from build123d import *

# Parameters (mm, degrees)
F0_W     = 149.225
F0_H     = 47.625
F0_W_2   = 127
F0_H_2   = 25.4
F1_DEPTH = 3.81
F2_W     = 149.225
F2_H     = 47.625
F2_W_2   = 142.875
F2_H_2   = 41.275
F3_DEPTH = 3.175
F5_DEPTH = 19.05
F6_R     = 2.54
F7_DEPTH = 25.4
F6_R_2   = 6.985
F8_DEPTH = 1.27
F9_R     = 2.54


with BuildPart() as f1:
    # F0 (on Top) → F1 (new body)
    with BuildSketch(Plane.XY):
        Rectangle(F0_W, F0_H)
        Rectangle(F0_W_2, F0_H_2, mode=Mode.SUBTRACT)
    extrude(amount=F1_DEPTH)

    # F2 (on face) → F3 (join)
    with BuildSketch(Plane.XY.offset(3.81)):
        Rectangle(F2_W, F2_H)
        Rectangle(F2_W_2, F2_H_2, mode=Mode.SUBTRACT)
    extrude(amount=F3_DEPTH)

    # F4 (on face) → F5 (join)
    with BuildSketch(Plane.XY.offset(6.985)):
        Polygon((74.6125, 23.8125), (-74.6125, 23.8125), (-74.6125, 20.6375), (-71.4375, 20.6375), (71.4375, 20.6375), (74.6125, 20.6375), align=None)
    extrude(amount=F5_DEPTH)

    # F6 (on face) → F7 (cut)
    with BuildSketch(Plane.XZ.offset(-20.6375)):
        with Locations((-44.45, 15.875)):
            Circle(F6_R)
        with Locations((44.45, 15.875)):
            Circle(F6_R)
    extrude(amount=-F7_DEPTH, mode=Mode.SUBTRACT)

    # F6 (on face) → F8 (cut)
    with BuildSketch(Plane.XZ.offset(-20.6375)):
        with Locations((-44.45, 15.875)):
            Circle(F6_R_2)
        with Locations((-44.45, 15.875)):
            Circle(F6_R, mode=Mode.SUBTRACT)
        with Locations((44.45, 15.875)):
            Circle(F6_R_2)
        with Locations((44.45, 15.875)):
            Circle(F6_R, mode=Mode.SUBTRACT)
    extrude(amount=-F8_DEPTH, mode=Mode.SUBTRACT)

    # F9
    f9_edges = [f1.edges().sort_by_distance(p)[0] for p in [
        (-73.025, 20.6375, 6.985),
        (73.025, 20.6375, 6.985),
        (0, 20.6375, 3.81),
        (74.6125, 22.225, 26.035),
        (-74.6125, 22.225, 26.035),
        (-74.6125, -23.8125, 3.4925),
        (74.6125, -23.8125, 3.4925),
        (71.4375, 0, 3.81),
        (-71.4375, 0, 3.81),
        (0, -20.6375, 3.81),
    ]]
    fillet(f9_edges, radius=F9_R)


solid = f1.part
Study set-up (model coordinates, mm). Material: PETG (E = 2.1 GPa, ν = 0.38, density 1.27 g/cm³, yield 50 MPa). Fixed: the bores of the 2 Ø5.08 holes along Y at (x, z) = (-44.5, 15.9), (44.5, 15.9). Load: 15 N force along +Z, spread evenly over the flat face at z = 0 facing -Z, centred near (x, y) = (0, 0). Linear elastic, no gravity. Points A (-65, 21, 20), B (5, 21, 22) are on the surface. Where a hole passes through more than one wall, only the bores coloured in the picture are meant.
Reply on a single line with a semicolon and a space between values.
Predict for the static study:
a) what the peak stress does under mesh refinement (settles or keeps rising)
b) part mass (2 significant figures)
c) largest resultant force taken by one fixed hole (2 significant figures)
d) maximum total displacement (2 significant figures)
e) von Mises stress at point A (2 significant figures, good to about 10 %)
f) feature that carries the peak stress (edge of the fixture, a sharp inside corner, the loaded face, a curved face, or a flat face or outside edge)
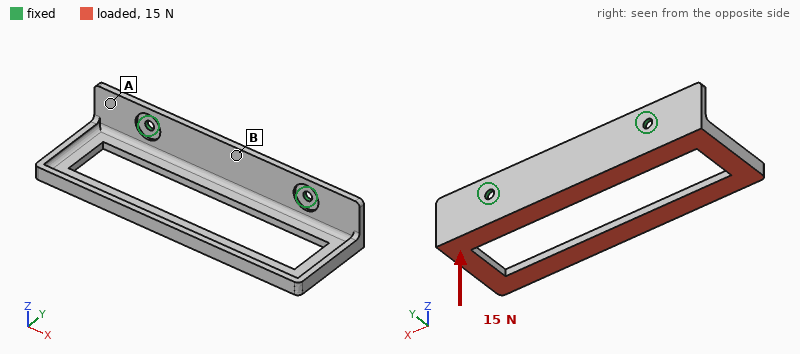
keeps rising; 35 g; 8.4 N; 1.6 mm; 1.2 MPa; edge of the fixture
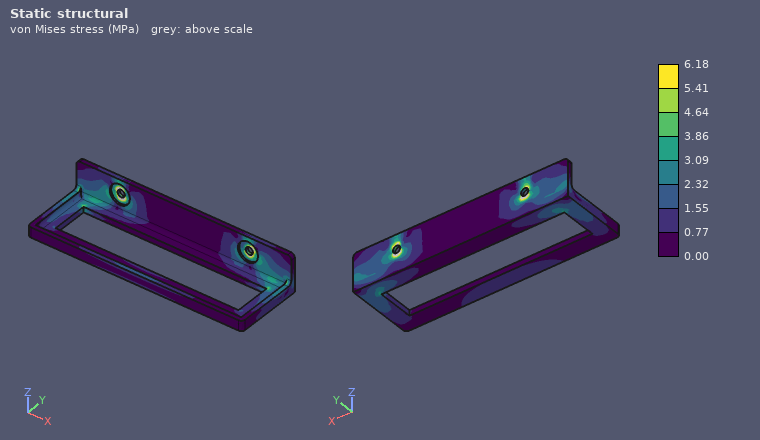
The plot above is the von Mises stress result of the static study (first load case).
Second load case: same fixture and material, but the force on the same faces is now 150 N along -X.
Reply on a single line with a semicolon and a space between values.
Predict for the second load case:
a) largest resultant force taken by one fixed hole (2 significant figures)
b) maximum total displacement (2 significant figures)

87 N; 1.7 mm
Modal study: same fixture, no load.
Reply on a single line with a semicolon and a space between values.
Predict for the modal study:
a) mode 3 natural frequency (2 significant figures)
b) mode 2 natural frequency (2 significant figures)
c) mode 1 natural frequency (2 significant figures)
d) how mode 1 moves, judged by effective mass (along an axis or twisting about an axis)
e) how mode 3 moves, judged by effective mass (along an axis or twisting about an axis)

340 Hz; 220 Hz; 110 Hz; along Z; along Y
